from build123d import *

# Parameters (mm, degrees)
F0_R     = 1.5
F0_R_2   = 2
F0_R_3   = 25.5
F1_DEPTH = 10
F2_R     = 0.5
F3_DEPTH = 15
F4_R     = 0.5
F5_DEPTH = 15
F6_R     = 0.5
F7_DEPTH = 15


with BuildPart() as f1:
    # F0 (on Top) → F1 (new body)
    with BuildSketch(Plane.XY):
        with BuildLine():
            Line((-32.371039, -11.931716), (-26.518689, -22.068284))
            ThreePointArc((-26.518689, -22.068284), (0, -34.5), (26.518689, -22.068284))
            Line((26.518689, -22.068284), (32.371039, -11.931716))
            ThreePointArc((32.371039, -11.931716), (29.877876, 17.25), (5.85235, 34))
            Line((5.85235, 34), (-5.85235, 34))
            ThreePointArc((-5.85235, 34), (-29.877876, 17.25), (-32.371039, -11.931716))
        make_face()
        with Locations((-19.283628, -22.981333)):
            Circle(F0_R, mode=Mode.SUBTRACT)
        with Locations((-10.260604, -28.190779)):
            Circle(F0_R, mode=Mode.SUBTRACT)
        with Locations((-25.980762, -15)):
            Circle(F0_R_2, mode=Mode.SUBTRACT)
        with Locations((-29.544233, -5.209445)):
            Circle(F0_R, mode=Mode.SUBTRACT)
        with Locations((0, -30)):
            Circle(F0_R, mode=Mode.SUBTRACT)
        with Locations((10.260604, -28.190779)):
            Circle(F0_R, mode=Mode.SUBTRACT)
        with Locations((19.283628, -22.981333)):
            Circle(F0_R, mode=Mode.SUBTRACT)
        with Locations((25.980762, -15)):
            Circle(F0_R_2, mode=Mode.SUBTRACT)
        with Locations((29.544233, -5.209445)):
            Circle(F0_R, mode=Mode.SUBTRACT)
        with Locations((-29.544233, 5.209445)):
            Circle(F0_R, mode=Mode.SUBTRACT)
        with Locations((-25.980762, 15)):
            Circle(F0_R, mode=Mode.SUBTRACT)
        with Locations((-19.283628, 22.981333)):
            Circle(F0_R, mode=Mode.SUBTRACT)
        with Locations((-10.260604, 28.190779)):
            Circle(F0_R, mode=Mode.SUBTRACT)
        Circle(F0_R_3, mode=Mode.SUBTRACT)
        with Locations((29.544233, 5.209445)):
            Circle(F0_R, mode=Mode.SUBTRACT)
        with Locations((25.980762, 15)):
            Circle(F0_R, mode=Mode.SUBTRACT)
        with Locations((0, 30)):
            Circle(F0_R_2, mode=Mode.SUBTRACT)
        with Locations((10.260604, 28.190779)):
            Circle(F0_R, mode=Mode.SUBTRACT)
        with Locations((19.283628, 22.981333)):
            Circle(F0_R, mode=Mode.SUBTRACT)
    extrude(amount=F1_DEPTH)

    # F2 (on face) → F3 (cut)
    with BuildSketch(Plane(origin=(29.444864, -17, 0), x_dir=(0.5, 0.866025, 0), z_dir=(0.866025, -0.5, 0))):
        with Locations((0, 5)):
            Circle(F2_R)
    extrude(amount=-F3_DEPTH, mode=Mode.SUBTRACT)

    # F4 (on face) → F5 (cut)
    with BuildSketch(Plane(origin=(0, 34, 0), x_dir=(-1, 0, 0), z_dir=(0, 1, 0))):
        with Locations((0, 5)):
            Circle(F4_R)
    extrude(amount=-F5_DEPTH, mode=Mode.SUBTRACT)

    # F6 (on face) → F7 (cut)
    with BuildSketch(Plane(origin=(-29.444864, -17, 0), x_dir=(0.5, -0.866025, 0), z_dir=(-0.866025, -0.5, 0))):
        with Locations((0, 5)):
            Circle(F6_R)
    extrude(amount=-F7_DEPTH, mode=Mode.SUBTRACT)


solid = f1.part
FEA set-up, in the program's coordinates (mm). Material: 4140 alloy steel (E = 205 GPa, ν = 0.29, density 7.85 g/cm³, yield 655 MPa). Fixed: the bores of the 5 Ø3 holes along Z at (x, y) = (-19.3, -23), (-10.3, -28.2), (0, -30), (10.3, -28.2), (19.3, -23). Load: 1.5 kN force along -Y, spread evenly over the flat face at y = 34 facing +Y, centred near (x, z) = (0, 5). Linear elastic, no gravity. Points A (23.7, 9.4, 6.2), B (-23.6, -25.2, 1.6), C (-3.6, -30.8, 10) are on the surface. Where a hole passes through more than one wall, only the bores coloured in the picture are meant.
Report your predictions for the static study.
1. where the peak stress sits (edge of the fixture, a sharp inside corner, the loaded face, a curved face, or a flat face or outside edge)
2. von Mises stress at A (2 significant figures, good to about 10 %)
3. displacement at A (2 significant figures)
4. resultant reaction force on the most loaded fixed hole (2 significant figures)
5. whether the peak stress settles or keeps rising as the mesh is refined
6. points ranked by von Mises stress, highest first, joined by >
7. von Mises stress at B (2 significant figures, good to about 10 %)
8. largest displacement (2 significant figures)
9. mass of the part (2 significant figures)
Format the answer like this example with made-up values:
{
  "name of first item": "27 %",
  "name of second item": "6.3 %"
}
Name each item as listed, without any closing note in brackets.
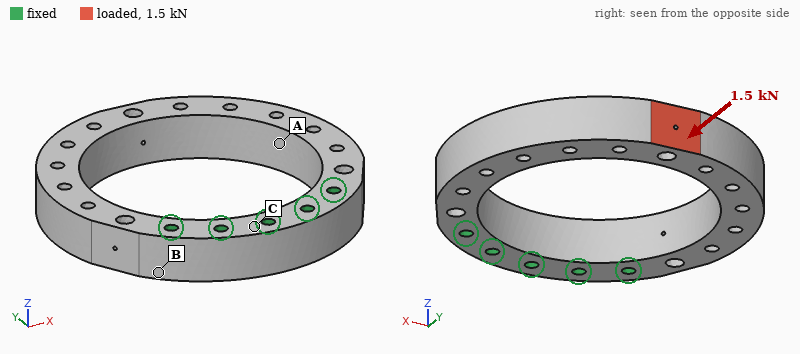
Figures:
{
  "where the peak stress sits": "a sharp inside corner",
  "von Mises stress at A": "60 MPa",
  "displacement at A": "15 µm",
  "resultant reaction force on the most loaded fixed hole": "1.1 kN",
  "whether the peak stress settles or keeps rising as the mesh is refined": "keeps rising",
  "points ranked by von Mises stress, highest first, joined by >": "A > B > C",
  "von Mises stress at B": "40 MPa",
  "largest displacement": "27 µm",
  "mass of the part": "120 g"
}
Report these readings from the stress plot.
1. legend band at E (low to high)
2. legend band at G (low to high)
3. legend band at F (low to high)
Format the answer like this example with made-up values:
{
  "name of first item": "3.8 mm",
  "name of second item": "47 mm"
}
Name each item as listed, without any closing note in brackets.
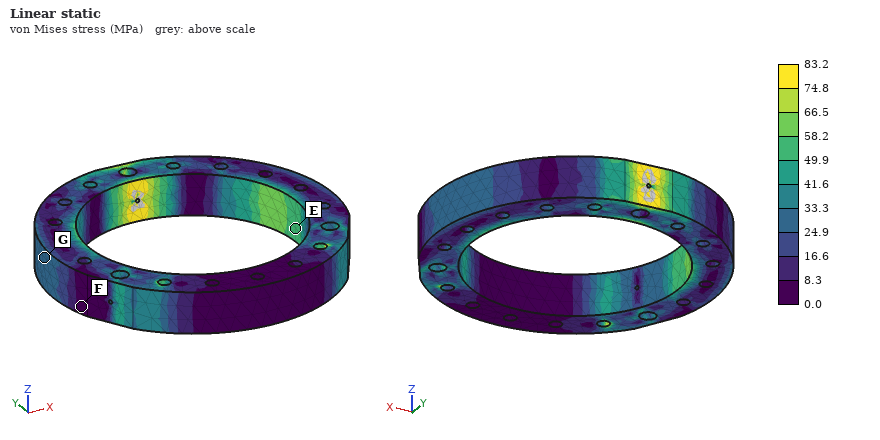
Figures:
{
  "legend band at E": "49.9 to 58.2 MPa",
  "legend band at G": "24.9 to 33.3 MPa",
  "legend band at F": "0.0 to 8.3 MPa"
}
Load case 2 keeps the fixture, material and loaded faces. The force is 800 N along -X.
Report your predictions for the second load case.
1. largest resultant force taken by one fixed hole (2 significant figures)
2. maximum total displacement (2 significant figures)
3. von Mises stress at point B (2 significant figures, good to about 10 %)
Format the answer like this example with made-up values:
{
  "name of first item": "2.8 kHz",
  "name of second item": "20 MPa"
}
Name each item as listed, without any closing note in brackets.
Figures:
{
  "largest resultant force taken by one fixed hole": "1.2 kN",
  "maximum total displacement": "60 µm",
  "von Mises stress at point B": "69 MPa"
}
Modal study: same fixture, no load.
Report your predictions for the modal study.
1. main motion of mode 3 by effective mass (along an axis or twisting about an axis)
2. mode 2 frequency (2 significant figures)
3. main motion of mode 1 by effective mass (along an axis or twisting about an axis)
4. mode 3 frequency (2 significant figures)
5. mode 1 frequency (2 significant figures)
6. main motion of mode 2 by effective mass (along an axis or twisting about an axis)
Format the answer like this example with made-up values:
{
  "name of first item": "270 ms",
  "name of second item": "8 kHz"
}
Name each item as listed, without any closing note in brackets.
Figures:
{
  "main motion of mode 3 by effective mass": "twisting about Y",
  "mode 2 frequency": "2600 Hz",
  "main motion of mode 1 by effective mass": "along Z",
  "mode 3 frequency": "4000 Hz",
  "mode 1 frequency": "1600 Hz",
  "main motion of mode 2 by effective mass": "along X"
}
